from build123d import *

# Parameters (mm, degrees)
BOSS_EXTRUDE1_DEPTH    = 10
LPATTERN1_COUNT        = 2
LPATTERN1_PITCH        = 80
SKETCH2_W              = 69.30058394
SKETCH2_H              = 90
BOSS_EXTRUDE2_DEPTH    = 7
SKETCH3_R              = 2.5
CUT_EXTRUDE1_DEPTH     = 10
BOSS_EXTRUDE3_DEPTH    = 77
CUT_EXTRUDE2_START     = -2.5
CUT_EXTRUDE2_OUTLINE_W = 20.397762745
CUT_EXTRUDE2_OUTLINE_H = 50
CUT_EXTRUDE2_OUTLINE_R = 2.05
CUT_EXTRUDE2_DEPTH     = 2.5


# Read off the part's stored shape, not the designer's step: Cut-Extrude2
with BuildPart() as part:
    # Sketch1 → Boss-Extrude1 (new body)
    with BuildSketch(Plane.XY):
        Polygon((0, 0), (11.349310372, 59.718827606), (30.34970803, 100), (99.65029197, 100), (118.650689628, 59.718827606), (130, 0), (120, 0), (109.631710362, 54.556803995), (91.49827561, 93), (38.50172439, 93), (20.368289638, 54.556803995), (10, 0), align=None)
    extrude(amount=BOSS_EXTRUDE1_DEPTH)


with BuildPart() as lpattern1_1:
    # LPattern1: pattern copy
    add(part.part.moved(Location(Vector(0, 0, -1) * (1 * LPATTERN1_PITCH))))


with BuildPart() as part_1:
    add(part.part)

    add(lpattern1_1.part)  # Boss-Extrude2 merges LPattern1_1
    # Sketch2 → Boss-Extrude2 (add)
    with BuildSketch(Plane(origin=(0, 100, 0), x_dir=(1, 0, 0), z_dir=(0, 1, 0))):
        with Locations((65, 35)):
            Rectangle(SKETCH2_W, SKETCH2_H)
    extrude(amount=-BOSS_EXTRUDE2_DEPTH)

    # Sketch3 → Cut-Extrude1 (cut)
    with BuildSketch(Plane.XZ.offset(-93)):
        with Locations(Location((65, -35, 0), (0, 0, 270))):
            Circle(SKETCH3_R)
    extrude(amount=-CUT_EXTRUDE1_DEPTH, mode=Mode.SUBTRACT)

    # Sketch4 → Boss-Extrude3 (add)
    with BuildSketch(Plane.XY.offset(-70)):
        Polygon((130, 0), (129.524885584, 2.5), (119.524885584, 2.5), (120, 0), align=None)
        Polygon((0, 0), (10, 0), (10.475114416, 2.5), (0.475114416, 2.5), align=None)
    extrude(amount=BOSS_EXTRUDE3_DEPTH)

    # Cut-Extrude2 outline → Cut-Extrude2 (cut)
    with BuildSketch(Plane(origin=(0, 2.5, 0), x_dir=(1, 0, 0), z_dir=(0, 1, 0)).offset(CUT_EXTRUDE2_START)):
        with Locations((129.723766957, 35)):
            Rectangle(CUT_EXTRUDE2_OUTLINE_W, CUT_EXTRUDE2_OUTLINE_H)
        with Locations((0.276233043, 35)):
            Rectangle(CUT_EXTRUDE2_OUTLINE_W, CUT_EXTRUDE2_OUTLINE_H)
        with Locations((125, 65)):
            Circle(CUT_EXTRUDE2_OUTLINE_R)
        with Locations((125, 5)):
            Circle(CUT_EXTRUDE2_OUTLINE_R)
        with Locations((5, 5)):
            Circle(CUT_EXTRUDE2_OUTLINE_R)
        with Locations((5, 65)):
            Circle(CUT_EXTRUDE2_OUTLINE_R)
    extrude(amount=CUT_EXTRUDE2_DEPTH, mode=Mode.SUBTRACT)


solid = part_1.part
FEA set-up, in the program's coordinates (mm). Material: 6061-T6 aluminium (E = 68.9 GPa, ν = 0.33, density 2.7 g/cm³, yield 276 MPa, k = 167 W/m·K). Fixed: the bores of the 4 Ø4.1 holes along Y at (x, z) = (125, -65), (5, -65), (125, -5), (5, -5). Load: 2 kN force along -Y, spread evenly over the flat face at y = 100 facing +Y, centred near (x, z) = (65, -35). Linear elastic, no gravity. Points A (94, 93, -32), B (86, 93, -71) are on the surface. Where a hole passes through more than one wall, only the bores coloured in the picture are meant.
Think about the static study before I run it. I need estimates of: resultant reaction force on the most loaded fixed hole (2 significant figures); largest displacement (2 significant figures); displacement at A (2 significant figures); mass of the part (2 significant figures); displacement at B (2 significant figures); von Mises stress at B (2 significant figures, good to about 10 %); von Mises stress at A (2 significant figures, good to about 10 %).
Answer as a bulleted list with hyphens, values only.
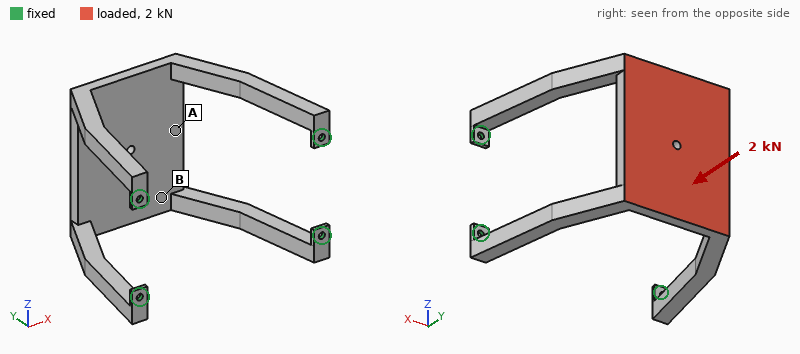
- 530 N
- 0.12 mm
- 0.11 mm
- 230 g
- 0.068 mm
- 11 MPa
- 25 MPa
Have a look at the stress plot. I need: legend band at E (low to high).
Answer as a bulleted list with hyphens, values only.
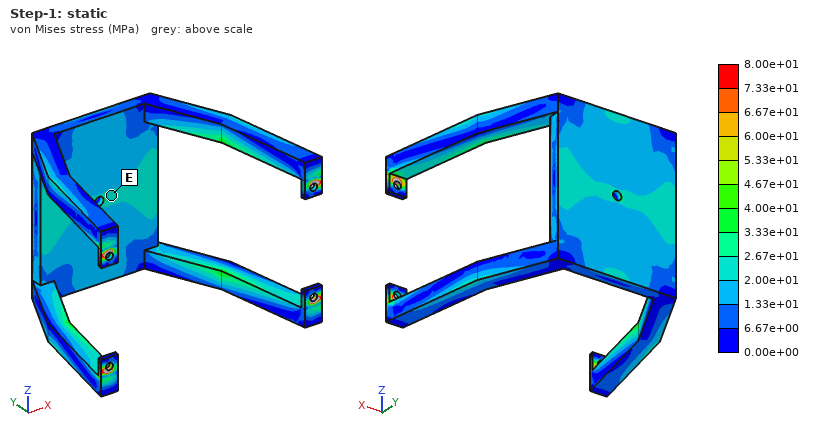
- 2.00e+01 to 2.67e+01 MPa
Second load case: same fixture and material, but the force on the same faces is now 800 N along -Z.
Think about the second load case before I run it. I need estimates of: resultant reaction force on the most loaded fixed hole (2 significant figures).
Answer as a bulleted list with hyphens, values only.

- 520 N
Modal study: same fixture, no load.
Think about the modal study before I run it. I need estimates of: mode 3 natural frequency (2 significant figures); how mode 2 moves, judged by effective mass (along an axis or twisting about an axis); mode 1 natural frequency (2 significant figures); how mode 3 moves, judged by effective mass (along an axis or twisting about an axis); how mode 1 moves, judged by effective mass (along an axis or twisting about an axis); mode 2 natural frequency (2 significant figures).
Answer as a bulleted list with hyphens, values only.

- 770 Hz
- along X
- 260 Hz
- twisting about Y
- along Z
- 530 Hz
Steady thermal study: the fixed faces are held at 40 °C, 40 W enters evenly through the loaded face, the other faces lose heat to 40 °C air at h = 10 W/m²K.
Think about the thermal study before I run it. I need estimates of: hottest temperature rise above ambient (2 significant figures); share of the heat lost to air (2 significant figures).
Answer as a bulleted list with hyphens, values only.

- 64 K
- 26 %
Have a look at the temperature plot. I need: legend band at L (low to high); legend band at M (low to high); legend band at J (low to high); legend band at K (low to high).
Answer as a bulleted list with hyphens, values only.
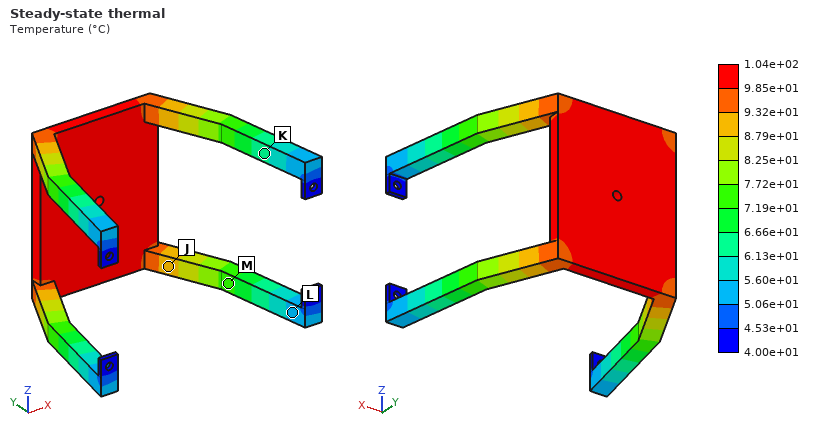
- 5.06e+01 to 5.60e+01 °C
- 7.19e+01 to 7.72e+01 °C
- 8.79e+01 to 9.32e+01 °C
- 6.13e+01 to 6.66e+01 °C
